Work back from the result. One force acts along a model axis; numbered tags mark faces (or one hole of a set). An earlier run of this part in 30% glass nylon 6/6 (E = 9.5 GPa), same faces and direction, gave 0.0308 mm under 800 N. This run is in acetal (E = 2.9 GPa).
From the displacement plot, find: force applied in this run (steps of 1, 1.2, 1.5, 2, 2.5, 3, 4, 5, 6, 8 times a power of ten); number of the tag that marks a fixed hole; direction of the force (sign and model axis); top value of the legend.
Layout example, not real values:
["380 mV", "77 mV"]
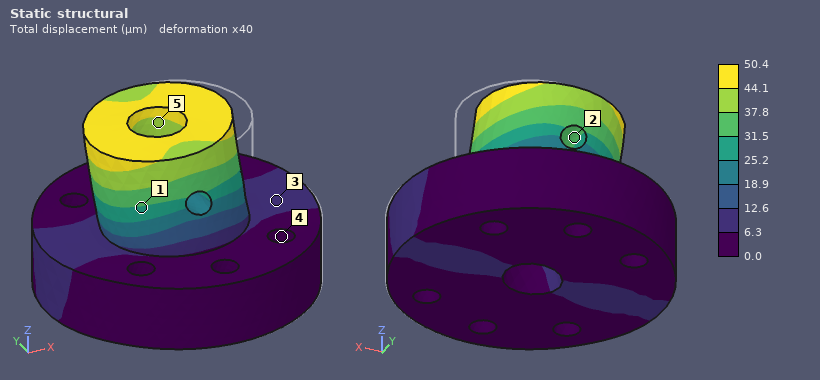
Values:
["400 N", "4", "-X", "50.4 µm"]
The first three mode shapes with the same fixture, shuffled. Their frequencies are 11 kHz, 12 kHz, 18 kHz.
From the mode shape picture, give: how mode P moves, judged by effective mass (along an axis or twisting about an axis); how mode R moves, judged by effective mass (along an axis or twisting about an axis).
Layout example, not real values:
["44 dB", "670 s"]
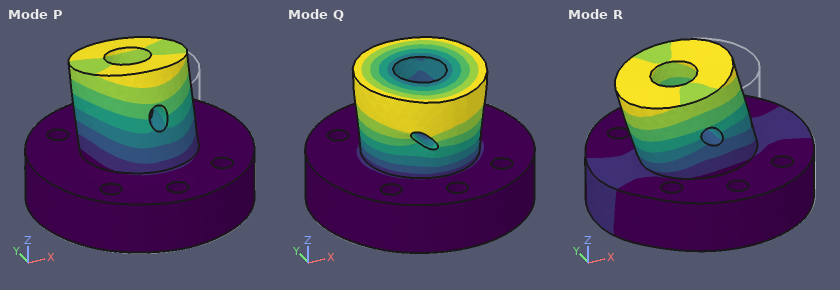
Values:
["along Y", "along X"]
